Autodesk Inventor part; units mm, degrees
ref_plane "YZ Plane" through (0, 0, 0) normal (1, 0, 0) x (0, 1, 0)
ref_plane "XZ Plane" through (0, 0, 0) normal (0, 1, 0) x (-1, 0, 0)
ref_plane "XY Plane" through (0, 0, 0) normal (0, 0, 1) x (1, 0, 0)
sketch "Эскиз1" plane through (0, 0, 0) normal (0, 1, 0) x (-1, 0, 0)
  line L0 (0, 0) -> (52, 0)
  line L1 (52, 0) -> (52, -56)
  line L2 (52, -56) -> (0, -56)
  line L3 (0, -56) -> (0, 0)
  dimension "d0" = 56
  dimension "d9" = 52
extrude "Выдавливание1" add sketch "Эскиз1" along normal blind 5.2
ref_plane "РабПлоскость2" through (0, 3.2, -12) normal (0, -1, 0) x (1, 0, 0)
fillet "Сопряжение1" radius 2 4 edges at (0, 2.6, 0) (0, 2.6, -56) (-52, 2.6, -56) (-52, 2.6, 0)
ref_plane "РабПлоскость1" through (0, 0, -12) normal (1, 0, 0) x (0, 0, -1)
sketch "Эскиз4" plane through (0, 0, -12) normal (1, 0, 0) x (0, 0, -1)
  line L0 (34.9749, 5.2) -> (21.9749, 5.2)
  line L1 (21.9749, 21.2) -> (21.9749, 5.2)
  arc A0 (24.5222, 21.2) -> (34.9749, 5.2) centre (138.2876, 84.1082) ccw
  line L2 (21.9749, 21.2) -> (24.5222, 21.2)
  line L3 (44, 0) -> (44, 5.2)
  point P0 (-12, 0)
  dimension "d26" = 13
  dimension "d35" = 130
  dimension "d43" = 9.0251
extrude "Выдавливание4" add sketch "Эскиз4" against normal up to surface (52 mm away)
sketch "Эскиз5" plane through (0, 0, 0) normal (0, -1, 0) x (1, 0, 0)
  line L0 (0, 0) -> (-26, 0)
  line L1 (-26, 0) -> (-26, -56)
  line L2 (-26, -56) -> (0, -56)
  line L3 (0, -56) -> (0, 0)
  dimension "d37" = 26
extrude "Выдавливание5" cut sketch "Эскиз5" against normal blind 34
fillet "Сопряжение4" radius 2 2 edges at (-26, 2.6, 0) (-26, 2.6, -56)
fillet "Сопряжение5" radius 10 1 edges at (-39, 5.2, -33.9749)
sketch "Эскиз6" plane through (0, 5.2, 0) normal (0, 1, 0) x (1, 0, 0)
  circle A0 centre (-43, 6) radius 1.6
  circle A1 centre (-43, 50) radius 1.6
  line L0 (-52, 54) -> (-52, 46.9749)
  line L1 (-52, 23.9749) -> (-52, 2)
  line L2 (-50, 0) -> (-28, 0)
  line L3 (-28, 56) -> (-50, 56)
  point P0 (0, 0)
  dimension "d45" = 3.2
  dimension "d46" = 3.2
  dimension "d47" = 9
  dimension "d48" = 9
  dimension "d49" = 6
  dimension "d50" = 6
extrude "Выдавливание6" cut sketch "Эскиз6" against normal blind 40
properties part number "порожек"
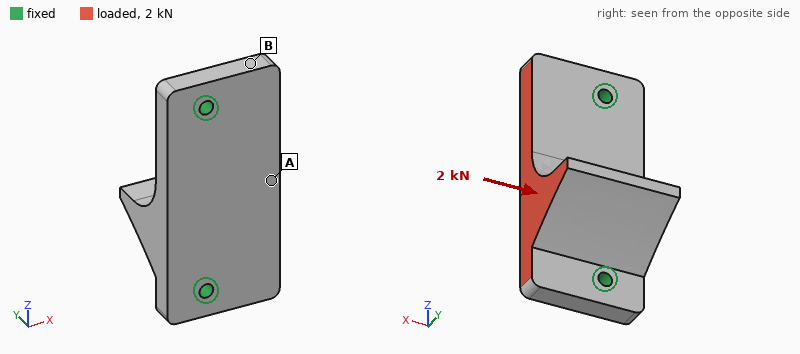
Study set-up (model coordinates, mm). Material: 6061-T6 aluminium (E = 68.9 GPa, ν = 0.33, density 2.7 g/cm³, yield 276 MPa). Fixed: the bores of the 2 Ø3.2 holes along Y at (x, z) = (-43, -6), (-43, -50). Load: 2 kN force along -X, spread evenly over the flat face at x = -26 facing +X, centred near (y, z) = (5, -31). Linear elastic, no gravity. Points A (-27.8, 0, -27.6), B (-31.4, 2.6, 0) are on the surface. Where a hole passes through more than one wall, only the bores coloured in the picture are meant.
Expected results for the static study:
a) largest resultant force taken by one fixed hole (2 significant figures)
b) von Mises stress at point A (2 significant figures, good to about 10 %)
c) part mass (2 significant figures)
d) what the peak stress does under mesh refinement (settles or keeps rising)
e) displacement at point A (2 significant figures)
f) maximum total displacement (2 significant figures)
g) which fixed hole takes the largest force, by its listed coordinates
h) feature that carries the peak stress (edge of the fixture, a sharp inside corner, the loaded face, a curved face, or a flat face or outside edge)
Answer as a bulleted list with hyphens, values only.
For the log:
- 1.2 kN
- 17 MPa
- 30 g
- keeps rising
- 17 µm
- 38 µm
- (-43, -50)
- edge of the fixture
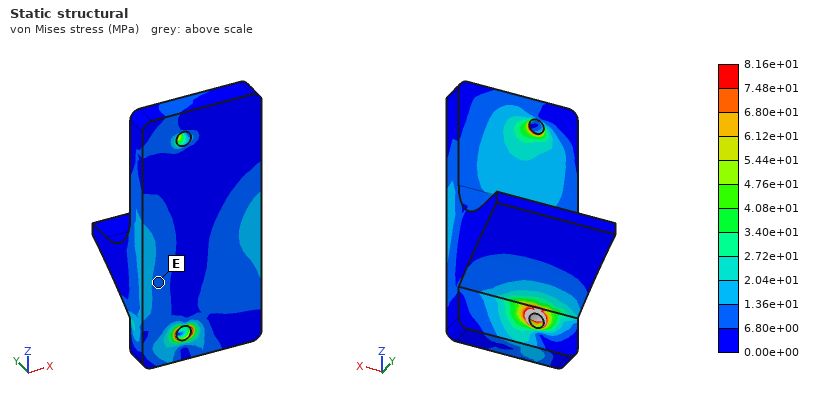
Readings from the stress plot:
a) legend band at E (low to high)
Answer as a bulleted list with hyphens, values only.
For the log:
- 6.80e+00 to 1.36e+01 MPa
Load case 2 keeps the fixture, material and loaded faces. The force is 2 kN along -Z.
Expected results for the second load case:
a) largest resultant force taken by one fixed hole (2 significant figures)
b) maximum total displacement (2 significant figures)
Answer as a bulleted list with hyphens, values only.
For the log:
- 1.3 kN
- 21 µm
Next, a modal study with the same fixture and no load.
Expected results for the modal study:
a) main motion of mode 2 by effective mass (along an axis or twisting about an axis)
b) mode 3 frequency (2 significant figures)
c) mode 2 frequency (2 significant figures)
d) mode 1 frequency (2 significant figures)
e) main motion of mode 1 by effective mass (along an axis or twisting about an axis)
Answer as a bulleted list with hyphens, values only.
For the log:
- along Y
- 16 kHz
- 9400 Hz
- 6400 Hz
- along Y
